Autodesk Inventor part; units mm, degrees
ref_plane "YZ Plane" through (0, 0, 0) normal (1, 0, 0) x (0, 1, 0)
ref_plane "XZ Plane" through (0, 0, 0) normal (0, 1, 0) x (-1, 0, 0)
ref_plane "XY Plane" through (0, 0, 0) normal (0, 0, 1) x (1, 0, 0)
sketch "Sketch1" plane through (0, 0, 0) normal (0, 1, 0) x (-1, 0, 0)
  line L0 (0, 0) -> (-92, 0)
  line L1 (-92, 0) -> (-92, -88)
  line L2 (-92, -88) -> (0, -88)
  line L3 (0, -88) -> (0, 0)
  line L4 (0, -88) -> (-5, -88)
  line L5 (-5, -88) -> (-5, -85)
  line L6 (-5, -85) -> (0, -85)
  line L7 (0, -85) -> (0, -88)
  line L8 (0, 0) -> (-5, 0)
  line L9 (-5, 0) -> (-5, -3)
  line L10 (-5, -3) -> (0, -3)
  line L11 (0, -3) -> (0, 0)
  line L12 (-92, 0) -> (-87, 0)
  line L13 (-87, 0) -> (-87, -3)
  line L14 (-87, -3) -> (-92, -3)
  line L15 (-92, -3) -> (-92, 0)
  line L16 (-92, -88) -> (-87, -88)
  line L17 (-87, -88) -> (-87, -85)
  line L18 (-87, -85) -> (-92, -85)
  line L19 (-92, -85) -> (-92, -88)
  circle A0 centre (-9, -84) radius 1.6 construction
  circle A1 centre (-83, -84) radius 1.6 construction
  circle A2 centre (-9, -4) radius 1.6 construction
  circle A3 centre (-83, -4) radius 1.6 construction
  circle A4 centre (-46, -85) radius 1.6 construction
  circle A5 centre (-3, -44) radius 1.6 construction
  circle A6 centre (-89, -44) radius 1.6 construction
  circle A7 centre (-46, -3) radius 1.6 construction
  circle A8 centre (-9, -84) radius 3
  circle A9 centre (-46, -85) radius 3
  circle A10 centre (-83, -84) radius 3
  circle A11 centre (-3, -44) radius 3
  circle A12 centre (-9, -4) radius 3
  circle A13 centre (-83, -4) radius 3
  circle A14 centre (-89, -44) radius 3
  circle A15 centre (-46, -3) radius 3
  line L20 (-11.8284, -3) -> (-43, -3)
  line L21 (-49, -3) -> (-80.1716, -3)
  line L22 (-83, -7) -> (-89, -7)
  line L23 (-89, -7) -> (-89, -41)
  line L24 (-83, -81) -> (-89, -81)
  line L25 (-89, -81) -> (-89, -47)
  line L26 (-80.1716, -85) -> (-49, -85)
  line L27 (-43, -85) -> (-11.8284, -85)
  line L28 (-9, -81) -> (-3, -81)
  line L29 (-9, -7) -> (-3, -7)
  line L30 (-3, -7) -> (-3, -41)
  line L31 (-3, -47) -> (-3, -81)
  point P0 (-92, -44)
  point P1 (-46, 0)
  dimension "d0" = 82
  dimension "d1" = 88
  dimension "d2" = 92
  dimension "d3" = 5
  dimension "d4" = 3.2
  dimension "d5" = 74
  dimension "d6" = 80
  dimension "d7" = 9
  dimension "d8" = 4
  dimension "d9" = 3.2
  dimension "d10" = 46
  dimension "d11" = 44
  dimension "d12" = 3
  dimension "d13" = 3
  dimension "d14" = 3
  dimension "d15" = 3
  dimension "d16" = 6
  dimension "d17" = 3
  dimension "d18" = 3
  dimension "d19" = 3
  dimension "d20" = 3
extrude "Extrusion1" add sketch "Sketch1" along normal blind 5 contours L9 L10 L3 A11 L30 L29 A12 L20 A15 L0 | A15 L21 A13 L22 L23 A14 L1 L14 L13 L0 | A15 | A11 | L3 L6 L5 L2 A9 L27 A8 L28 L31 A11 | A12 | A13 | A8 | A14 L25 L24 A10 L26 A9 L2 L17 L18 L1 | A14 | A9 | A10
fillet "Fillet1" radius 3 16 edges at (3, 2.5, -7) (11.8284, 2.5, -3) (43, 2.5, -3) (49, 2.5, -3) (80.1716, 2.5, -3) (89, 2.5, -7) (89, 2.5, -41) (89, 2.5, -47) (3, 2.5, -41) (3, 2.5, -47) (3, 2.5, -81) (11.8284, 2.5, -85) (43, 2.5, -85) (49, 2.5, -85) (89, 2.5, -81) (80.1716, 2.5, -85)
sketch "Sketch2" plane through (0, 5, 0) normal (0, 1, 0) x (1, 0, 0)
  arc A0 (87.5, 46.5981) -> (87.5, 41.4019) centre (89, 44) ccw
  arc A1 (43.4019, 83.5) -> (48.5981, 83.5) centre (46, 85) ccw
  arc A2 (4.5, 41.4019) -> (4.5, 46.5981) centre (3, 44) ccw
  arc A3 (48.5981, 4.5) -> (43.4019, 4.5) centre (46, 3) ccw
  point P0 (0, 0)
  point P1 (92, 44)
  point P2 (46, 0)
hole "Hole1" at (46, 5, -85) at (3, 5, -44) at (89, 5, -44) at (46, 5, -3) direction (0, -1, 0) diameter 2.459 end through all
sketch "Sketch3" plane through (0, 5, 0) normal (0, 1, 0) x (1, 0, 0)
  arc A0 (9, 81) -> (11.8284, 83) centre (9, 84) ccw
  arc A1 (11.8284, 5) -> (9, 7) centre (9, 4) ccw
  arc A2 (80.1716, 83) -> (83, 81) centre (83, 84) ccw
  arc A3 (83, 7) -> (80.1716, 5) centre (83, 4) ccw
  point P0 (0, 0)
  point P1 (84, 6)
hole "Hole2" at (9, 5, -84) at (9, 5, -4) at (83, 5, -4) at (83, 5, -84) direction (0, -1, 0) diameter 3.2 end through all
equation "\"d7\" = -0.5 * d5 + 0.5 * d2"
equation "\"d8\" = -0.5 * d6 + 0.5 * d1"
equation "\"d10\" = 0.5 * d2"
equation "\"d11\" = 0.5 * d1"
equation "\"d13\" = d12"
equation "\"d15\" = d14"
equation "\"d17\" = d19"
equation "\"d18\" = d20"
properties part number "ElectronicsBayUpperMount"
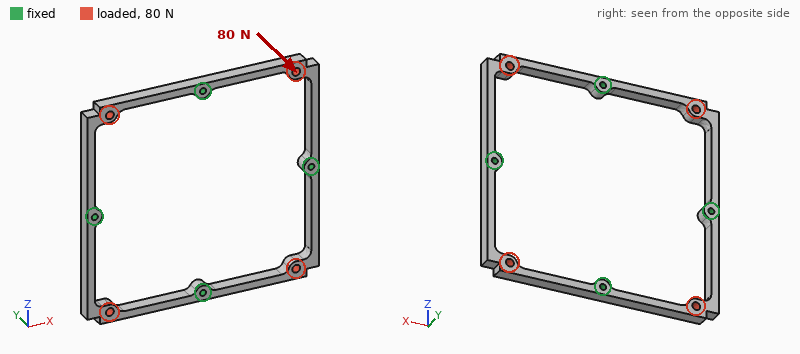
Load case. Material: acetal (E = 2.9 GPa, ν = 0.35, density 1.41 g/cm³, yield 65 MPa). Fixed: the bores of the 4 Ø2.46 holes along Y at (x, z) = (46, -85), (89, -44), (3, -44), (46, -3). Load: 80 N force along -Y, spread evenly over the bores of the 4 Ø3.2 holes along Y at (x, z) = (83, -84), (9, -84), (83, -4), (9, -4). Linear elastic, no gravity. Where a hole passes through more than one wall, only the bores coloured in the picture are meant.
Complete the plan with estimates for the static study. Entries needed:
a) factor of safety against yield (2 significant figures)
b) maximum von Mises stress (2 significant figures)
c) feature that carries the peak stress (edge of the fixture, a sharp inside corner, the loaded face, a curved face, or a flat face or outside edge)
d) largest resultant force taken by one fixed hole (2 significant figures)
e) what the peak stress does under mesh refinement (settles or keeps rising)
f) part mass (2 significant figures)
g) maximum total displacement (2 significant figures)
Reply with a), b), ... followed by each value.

a) 2.4
b) 28 MPa
c) a curved face
d) 22 N
e) settles
f) 8.1 g
g) 1.4 mm
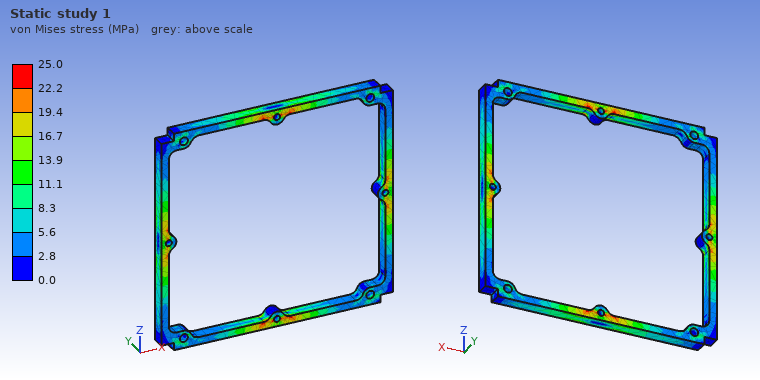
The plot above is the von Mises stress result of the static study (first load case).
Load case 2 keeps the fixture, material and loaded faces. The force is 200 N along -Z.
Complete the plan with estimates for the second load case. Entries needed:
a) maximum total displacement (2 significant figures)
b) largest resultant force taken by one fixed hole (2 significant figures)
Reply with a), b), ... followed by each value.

a) 0.36 mm
b) 84 N
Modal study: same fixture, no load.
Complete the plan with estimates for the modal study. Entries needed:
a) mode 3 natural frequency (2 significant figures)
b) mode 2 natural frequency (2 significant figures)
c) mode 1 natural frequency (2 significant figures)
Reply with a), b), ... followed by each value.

a) 700 Hz
b) 700 Hz
c) 700 Hz
